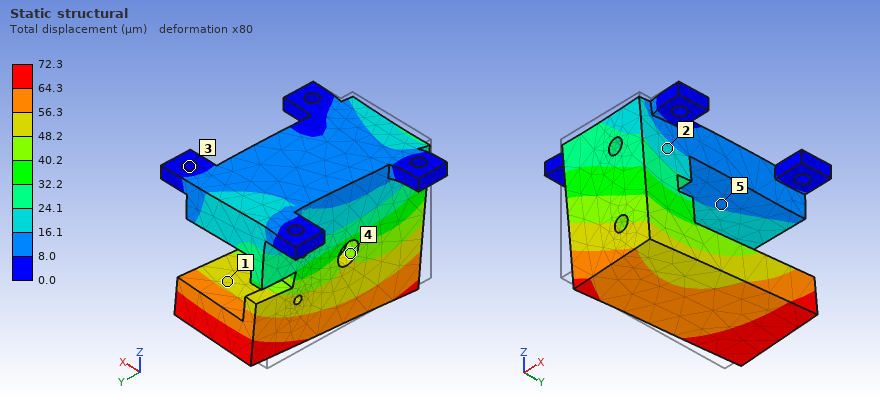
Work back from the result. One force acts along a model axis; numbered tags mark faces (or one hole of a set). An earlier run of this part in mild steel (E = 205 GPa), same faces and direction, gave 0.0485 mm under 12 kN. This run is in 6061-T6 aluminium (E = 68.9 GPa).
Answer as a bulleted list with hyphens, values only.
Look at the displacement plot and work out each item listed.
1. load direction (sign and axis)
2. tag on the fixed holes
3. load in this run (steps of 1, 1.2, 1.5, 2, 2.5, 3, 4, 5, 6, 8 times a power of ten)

- +Y
- 3
- 6 kN
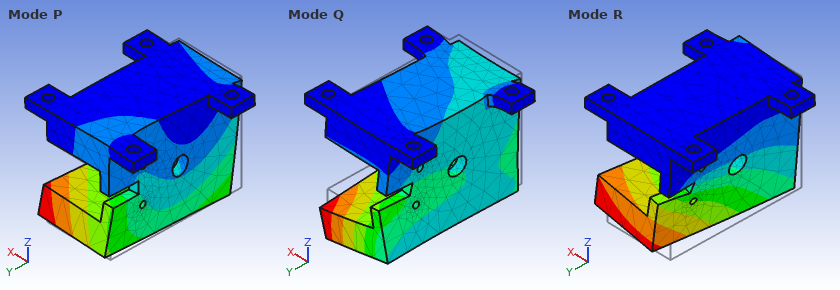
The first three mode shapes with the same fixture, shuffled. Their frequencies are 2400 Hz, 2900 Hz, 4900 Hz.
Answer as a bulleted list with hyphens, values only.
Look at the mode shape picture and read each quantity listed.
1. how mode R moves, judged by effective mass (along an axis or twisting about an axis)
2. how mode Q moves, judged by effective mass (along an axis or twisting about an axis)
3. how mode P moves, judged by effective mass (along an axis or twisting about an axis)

- along X
- along Z
- along Y
